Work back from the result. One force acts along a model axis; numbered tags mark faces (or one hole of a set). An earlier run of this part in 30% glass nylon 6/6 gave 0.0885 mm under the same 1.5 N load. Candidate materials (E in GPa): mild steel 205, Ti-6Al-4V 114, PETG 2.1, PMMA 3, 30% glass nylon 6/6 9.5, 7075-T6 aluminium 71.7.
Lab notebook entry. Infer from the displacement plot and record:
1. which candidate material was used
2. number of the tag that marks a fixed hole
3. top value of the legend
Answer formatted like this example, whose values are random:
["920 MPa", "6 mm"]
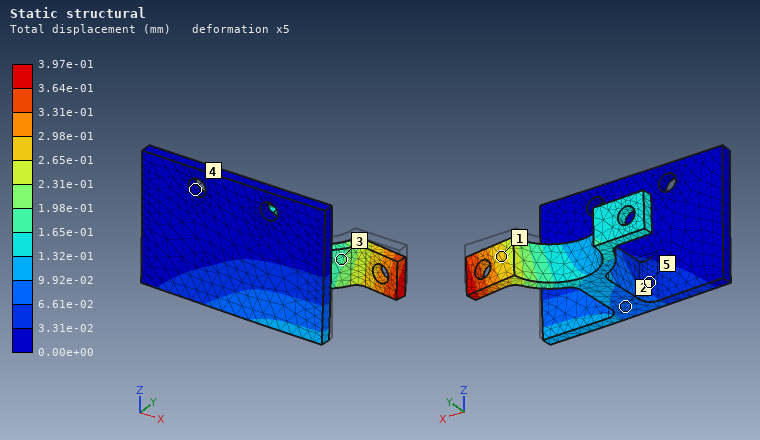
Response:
["PETG", "4", "3.97e-01 mm"]
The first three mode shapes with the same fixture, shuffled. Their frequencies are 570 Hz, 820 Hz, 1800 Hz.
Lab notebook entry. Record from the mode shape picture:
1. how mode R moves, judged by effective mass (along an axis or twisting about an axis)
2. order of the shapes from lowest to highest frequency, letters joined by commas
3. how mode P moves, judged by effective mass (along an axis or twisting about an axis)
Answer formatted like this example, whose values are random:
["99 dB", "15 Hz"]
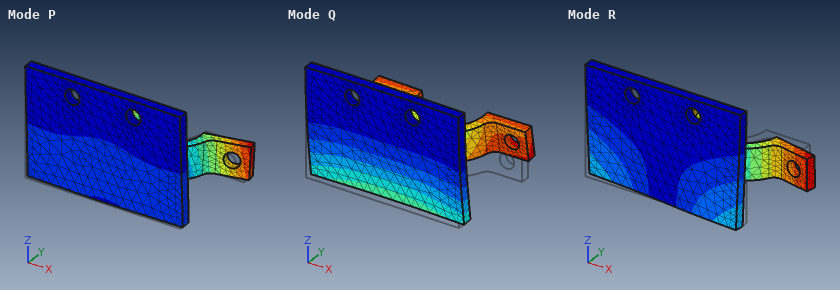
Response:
["along X", "Q, R, P", "along Y"]
